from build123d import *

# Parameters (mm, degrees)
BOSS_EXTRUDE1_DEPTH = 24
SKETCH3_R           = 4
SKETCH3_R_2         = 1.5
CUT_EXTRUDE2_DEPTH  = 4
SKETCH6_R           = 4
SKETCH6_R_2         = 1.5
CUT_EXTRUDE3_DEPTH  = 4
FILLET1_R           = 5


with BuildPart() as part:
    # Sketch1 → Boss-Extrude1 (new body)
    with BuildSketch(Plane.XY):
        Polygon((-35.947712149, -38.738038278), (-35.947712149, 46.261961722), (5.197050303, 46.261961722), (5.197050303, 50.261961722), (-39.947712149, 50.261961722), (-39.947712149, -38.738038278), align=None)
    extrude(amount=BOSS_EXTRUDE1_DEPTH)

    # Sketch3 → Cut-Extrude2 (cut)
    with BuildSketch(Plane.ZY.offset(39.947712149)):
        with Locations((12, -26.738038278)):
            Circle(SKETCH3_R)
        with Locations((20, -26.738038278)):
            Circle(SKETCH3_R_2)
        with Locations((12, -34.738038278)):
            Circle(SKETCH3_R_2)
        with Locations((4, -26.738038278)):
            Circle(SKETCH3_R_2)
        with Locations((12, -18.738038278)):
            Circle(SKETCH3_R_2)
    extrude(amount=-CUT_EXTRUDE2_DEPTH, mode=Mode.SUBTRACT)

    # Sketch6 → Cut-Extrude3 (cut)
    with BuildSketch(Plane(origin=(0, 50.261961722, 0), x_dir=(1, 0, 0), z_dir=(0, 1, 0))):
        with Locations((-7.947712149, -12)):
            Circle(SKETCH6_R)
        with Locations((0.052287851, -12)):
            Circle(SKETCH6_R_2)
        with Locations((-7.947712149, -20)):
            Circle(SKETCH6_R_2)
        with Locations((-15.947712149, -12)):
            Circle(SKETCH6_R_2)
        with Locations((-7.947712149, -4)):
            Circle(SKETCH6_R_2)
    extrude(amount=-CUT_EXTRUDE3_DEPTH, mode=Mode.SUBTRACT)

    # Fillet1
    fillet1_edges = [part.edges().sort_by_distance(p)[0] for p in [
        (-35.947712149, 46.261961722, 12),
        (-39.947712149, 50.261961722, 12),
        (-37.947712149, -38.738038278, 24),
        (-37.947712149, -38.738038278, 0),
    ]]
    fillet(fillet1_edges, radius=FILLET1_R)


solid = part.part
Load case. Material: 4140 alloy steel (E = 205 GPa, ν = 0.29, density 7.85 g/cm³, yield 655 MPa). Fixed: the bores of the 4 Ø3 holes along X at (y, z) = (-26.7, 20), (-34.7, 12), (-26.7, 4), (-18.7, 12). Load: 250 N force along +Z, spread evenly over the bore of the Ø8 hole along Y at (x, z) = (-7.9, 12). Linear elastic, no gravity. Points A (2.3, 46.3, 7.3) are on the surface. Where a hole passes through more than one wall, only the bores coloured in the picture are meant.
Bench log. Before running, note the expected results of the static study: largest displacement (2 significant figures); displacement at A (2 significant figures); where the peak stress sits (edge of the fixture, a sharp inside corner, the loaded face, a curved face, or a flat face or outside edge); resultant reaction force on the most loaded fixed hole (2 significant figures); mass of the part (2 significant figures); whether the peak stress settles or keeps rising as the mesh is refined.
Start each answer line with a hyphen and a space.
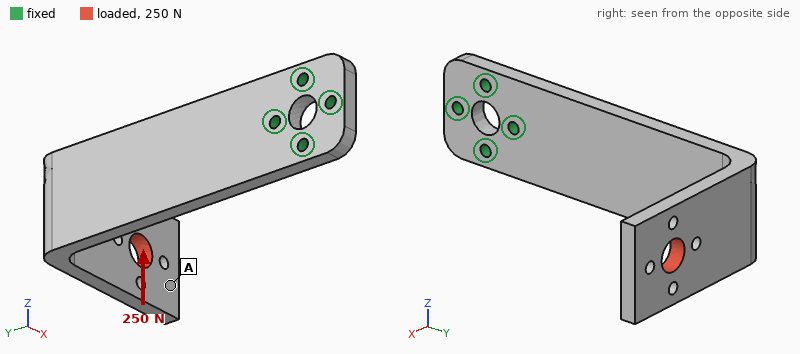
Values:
- 0.60 mm
- 0.55 mm
- edge of the fixture
- 830 N
- 93 g
- keeps rising
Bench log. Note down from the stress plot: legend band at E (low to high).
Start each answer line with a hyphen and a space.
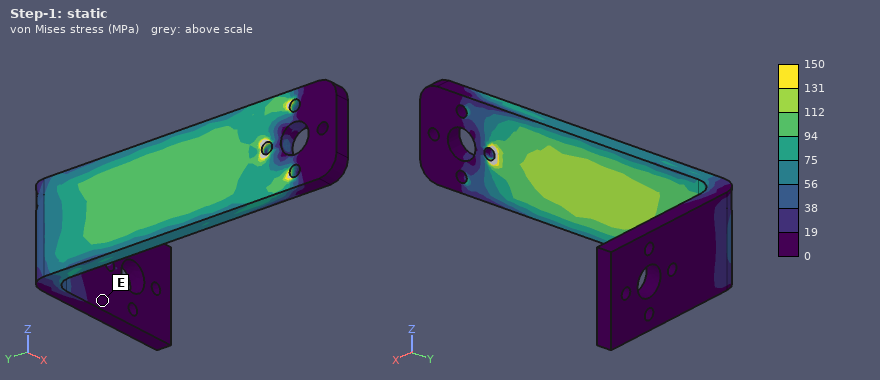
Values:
- 0 to 19 MPa
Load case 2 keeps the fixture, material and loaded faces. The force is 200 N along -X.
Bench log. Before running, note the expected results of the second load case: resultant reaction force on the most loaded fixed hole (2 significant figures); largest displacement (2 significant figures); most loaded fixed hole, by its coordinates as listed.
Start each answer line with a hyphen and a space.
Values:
- 990 N
- 1.1 mm
- (-18.7, 12)
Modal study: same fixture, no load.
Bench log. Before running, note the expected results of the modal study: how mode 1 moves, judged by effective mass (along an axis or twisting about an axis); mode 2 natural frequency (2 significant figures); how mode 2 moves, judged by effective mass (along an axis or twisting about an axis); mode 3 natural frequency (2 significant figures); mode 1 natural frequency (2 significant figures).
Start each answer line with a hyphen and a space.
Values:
- along X
- 820 Hz
- along Z
- 1300 Hz
- 360 Hz
